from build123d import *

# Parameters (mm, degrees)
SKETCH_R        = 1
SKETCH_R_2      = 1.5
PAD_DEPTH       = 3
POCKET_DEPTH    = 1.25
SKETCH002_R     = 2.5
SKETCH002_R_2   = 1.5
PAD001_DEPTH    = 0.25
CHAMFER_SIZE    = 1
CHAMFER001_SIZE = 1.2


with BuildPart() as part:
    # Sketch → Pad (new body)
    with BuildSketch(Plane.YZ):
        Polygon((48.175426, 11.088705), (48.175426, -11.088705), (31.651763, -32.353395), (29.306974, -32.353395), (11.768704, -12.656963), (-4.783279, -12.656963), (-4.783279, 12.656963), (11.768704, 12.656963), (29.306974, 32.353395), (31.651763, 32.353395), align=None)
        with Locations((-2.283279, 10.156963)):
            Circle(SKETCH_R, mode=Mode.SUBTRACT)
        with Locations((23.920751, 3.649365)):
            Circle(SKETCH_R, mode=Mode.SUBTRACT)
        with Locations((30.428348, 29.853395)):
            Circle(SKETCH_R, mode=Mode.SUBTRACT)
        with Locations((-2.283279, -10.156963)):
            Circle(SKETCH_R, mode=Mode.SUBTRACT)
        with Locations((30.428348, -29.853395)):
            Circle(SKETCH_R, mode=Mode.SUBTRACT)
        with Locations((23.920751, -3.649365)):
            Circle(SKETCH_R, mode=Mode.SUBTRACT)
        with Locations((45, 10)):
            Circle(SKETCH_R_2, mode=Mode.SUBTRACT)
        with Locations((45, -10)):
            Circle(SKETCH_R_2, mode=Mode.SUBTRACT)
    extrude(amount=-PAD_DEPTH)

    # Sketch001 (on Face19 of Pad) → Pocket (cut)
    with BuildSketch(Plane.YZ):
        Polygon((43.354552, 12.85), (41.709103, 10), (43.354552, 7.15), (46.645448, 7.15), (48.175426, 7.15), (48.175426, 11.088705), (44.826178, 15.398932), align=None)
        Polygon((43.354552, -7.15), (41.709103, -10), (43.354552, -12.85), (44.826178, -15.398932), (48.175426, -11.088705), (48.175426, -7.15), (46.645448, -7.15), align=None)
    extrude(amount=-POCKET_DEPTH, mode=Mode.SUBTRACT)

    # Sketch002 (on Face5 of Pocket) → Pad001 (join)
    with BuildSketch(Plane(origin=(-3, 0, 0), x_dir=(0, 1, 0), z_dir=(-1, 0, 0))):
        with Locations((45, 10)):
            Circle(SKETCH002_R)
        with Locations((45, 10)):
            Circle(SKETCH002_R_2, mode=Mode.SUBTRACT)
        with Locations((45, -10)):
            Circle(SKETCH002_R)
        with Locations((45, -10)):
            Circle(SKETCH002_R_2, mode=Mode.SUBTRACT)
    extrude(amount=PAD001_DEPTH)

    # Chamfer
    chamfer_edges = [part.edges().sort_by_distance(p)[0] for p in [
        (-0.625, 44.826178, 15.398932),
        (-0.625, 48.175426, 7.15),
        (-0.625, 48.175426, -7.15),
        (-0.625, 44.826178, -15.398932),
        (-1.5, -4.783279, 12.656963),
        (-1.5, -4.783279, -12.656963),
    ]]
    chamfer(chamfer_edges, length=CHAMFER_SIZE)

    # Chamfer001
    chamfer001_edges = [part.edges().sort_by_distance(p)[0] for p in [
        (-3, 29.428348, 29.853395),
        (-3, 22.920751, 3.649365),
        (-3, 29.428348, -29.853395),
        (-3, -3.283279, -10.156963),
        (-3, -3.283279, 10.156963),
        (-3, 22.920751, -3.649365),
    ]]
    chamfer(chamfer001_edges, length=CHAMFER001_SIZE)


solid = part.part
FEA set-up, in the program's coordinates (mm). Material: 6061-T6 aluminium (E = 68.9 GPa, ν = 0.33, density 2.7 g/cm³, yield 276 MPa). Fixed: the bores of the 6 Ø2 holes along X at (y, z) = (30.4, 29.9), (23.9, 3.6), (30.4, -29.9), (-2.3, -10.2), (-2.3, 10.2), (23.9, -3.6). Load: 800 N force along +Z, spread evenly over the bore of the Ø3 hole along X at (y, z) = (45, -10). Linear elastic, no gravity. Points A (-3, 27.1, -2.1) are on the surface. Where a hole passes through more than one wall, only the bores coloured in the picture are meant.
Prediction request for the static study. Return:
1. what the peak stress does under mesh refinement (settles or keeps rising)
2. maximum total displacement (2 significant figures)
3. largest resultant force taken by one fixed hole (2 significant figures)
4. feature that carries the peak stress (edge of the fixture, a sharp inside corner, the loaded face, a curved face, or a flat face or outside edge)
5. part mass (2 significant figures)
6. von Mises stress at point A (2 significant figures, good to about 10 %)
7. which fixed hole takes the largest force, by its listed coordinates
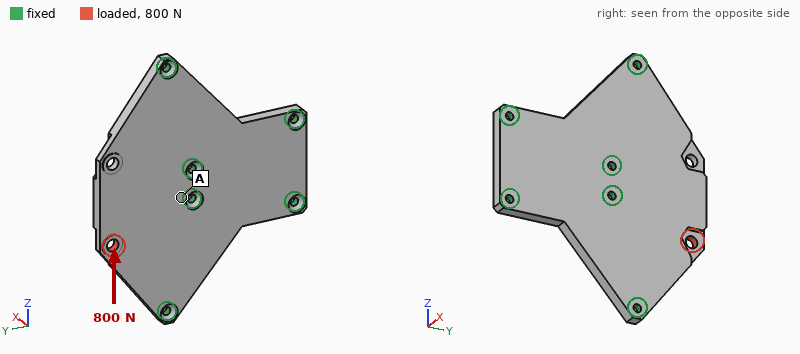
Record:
keeps rising
14 µm
370 N
edge of the fixture
16 g
8.9 MPa
(30.4, -29.9)
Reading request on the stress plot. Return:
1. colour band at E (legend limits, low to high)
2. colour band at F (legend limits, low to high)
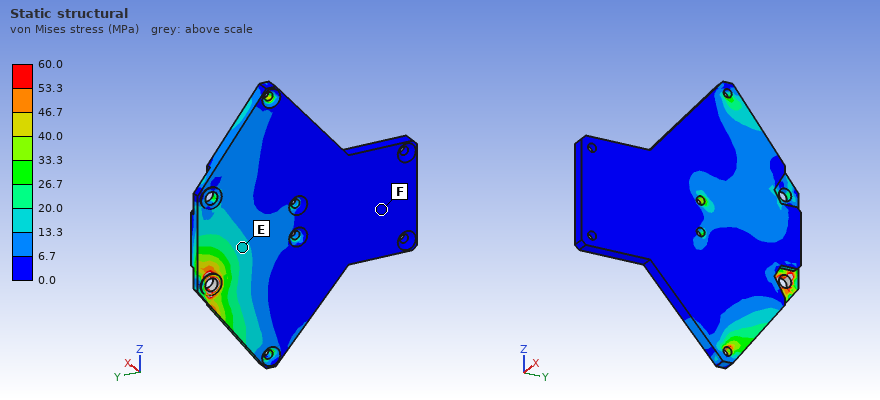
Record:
13.3 to 20.0 MPa
0.0 to 6.7 MPa
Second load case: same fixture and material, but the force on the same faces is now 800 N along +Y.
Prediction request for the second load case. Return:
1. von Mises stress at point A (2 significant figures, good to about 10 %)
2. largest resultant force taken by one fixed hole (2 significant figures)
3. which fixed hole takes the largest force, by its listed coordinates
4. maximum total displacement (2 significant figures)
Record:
20 MPa
340 N
(23.9, -3.6)
47 µm
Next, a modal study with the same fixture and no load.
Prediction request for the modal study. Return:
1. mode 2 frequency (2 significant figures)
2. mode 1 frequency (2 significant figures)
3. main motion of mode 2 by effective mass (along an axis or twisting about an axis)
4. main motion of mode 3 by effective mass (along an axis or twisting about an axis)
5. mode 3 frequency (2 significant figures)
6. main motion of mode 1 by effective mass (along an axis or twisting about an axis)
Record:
9400 Hz
4600 Hz
twisting about Y
along X
14 kHz
along X
